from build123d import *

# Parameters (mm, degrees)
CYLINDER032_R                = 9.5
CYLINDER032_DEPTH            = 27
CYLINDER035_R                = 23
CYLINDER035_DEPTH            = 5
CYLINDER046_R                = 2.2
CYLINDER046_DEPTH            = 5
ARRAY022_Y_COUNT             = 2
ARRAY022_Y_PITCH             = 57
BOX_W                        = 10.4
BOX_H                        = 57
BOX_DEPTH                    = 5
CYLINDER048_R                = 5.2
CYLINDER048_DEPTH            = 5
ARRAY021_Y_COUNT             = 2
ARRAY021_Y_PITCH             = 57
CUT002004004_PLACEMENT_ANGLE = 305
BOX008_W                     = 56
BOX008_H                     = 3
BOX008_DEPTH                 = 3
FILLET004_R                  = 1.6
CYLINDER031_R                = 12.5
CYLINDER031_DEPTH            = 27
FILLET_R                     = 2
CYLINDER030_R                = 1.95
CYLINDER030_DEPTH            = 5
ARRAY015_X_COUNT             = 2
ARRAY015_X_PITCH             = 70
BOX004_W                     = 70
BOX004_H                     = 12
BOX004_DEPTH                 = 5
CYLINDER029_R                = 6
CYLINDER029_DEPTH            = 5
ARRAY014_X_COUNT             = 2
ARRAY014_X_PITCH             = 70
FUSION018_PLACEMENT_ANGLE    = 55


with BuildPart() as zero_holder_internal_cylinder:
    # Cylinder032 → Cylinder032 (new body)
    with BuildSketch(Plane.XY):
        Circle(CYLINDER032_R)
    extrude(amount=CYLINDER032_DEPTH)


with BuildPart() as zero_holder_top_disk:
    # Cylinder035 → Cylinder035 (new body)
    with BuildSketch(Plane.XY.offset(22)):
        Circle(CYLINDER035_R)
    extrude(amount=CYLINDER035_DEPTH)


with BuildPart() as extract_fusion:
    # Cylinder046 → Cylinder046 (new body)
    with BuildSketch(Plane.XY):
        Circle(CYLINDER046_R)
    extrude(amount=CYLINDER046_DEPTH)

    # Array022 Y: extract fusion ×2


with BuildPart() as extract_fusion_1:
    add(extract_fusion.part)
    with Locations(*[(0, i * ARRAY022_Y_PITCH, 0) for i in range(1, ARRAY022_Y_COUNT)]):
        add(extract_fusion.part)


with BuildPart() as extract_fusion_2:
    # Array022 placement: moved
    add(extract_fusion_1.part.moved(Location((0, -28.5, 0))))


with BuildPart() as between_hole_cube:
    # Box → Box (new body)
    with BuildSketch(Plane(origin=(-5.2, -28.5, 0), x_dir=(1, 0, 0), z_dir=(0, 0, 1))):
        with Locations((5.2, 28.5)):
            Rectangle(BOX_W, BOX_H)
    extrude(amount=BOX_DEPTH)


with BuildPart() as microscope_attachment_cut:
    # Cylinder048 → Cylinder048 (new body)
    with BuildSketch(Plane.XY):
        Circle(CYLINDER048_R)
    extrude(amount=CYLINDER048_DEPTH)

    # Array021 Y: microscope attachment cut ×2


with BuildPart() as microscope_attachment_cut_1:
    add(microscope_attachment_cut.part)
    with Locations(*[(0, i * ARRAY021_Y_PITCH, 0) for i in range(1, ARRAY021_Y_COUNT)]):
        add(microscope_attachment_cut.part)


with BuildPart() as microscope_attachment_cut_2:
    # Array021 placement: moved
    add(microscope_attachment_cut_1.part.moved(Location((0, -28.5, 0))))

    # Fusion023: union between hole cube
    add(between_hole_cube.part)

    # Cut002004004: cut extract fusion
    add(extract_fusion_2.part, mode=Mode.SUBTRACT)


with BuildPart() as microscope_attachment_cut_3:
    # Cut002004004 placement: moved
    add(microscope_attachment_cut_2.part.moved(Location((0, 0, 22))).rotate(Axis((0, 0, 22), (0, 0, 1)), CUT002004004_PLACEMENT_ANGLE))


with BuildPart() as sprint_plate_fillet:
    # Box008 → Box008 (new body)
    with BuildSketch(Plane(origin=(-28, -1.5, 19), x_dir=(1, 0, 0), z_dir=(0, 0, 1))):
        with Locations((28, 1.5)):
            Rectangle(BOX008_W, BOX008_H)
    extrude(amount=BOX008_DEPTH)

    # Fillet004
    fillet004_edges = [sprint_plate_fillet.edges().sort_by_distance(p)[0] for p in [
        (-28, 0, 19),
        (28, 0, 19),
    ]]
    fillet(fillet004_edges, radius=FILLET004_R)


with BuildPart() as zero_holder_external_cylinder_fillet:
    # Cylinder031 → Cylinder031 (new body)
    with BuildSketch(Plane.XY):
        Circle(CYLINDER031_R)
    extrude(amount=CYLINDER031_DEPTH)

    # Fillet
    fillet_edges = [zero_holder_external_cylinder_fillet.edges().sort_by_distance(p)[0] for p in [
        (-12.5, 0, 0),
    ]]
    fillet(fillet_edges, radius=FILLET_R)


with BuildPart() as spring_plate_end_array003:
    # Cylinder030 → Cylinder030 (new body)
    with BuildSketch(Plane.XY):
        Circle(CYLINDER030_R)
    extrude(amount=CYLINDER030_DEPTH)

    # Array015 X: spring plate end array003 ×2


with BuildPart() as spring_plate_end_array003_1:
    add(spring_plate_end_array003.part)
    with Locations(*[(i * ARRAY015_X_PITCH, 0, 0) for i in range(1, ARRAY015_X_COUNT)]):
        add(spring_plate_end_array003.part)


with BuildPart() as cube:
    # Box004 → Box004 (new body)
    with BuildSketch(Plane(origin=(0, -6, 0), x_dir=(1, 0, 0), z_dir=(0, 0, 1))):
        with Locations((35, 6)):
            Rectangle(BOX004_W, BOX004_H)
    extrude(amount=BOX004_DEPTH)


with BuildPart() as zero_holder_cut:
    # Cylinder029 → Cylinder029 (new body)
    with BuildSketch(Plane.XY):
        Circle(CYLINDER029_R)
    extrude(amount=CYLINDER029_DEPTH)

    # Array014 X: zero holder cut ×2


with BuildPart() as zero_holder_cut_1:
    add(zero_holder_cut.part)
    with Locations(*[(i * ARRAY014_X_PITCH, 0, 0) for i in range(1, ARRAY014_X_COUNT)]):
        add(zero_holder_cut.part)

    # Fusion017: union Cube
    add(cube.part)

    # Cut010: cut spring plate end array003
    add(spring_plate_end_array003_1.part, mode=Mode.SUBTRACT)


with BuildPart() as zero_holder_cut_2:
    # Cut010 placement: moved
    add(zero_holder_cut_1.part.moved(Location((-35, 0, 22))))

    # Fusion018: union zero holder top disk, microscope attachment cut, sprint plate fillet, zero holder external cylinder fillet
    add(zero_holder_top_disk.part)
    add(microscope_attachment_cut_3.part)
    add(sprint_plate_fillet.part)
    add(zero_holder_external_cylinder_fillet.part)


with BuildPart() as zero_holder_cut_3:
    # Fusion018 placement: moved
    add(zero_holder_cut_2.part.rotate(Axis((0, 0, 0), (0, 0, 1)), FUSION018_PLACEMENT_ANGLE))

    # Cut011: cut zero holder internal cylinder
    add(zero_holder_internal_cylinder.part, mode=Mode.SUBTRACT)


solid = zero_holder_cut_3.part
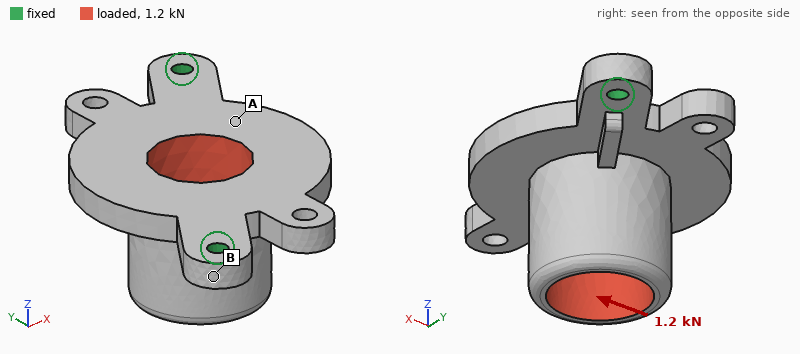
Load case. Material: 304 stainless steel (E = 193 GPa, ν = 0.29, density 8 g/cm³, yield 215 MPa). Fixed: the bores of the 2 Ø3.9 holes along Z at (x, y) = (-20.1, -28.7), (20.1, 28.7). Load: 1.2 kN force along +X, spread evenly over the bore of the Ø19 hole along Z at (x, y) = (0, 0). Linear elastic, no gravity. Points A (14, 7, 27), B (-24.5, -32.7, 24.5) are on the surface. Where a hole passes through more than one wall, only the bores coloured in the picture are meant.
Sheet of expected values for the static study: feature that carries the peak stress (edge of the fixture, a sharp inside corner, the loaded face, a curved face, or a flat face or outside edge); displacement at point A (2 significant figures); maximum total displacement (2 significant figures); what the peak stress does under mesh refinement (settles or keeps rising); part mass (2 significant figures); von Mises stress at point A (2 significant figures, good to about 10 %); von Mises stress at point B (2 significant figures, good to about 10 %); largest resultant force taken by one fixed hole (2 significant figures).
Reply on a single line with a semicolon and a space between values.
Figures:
edge of the fixture; 24 µm; 88 µm; keeps rising; 120 g; 23 MPa; 14 MPa; 620 N
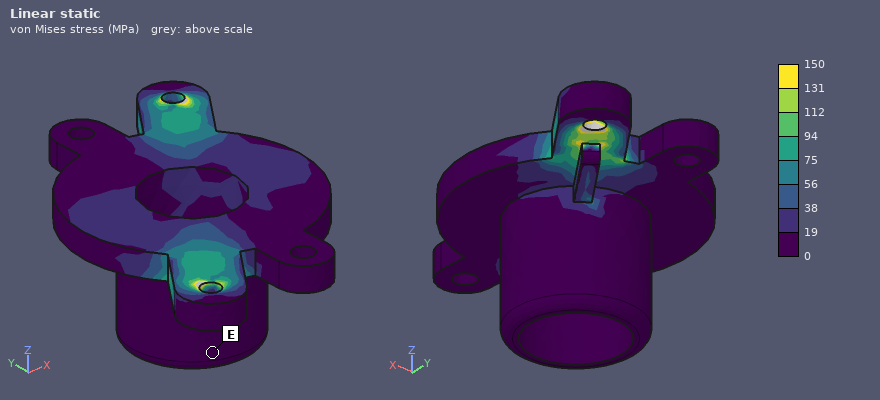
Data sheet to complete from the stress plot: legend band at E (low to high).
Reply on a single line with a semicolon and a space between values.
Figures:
0 to 19 MPa
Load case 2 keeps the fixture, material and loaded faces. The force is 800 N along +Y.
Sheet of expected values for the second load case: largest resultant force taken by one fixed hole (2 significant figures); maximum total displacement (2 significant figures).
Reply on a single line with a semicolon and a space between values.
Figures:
420 N; 41 µm
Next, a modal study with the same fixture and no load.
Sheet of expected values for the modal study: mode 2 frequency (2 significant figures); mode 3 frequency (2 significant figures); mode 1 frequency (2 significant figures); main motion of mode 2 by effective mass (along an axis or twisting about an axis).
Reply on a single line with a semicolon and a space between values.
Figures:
3500 Hz; 6900 Hz; 2100 Hz; along Z
